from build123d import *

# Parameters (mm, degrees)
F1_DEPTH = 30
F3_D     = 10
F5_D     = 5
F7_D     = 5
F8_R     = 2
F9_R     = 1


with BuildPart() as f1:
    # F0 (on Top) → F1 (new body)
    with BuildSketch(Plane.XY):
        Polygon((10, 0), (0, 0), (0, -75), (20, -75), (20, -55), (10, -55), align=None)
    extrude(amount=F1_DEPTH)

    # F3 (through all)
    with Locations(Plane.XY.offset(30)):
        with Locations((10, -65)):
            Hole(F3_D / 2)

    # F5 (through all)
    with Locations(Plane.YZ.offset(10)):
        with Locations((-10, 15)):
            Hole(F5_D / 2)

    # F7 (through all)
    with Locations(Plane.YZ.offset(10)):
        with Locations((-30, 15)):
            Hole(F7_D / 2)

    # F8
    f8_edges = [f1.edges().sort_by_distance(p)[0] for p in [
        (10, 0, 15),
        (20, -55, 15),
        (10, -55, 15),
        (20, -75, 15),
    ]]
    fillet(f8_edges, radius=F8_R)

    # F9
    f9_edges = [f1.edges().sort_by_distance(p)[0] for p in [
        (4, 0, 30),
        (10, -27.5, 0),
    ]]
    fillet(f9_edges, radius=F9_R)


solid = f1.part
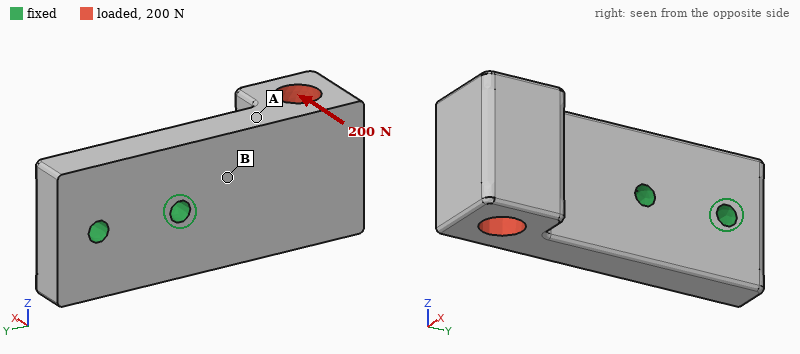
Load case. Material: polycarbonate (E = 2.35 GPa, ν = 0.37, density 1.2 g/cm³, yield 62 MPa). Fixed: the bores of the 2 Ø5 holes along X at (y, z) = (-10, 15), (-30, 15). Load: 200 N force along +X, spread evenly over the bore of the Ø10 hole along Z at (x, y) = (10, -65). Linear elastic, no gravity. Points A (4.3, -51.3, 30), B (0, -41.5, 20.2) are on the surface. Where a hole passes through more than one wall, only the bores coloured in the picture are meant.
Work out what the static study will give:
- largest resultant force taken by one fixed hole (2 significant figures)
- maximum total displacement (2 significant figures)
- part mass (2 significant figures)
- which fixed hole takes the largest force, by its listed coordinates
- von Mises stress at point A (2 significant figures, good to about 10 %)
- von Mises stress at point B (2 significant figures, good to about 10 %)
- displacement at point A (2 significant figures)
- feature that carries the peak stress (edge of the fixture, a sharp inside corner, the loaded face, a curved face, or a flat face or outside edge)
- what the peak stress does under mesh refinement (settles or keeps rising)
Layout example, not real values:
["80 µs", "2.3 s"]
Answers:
["320 N", "0.84 mm", "31 g", "(-30, 15)", "3.1 MPa", "8.7 MPa", "0.25 mm", "edge of the fixture", "keeps rising"]
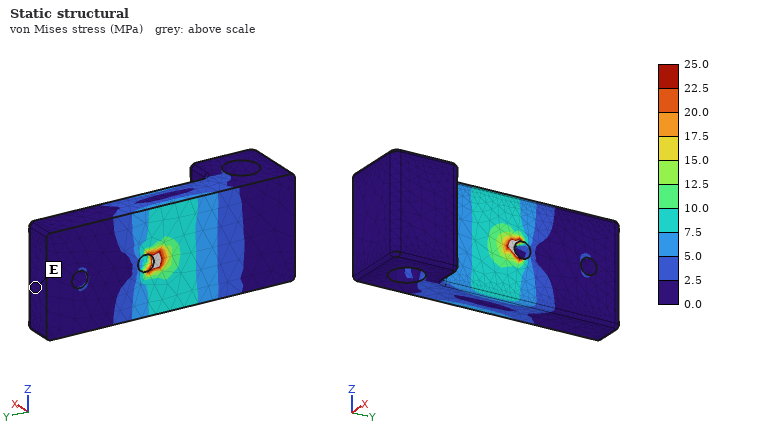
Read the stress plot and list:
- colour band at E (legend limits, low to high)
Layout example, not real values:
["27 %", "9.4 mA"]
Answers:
["0.0 to 2.5 MPa"]
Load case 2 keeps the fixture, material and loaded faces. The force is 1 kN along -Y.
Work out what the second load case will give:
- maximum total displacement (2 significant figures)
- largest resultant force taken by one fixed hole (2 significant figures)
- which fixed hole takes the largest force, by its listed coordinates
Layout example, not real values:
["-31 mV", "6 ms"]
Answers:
["0.91 mm", "790 N", "(-30, 15)"]
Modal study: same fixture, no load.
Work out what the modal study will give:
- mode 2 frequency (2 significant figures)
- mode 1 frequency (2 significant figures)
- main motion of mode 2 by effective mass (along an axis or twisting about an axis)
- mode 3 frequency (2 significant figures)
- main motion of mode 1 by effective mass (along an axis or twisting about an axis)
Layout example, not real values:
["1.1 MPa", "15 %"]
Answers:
["1400 Hz", "800 Hz", "along Z", "2100 Hz", "along X"]
